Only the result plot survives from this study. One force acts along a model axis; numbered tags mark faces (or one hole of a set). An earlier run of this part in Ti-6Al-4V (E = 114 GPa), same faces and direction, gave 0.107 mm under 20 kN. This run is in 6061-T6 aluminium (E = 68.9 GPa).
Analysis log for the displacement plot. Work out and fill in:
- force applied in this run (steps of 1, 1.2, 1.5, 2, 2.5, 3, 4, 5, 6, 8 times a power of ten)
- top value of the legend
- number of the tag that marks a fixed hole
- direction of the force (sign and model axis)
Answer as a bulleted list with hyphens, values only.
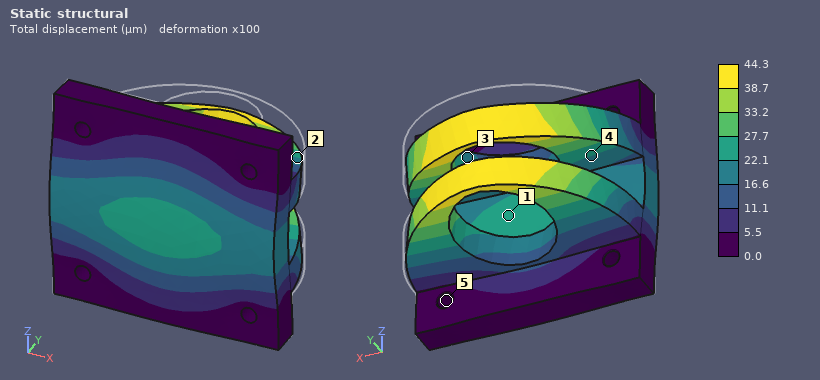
- 5 kN
- 44.3 µm
- 5
- -Y
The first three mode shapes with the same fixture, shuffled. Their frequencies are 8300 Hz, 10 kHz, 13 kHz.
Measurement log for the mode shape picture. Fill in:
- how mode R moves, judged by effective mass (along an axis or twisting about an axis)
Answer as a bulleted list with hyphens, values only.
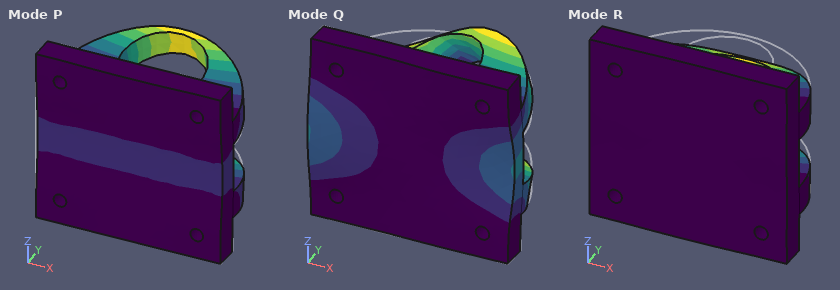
- along Z
